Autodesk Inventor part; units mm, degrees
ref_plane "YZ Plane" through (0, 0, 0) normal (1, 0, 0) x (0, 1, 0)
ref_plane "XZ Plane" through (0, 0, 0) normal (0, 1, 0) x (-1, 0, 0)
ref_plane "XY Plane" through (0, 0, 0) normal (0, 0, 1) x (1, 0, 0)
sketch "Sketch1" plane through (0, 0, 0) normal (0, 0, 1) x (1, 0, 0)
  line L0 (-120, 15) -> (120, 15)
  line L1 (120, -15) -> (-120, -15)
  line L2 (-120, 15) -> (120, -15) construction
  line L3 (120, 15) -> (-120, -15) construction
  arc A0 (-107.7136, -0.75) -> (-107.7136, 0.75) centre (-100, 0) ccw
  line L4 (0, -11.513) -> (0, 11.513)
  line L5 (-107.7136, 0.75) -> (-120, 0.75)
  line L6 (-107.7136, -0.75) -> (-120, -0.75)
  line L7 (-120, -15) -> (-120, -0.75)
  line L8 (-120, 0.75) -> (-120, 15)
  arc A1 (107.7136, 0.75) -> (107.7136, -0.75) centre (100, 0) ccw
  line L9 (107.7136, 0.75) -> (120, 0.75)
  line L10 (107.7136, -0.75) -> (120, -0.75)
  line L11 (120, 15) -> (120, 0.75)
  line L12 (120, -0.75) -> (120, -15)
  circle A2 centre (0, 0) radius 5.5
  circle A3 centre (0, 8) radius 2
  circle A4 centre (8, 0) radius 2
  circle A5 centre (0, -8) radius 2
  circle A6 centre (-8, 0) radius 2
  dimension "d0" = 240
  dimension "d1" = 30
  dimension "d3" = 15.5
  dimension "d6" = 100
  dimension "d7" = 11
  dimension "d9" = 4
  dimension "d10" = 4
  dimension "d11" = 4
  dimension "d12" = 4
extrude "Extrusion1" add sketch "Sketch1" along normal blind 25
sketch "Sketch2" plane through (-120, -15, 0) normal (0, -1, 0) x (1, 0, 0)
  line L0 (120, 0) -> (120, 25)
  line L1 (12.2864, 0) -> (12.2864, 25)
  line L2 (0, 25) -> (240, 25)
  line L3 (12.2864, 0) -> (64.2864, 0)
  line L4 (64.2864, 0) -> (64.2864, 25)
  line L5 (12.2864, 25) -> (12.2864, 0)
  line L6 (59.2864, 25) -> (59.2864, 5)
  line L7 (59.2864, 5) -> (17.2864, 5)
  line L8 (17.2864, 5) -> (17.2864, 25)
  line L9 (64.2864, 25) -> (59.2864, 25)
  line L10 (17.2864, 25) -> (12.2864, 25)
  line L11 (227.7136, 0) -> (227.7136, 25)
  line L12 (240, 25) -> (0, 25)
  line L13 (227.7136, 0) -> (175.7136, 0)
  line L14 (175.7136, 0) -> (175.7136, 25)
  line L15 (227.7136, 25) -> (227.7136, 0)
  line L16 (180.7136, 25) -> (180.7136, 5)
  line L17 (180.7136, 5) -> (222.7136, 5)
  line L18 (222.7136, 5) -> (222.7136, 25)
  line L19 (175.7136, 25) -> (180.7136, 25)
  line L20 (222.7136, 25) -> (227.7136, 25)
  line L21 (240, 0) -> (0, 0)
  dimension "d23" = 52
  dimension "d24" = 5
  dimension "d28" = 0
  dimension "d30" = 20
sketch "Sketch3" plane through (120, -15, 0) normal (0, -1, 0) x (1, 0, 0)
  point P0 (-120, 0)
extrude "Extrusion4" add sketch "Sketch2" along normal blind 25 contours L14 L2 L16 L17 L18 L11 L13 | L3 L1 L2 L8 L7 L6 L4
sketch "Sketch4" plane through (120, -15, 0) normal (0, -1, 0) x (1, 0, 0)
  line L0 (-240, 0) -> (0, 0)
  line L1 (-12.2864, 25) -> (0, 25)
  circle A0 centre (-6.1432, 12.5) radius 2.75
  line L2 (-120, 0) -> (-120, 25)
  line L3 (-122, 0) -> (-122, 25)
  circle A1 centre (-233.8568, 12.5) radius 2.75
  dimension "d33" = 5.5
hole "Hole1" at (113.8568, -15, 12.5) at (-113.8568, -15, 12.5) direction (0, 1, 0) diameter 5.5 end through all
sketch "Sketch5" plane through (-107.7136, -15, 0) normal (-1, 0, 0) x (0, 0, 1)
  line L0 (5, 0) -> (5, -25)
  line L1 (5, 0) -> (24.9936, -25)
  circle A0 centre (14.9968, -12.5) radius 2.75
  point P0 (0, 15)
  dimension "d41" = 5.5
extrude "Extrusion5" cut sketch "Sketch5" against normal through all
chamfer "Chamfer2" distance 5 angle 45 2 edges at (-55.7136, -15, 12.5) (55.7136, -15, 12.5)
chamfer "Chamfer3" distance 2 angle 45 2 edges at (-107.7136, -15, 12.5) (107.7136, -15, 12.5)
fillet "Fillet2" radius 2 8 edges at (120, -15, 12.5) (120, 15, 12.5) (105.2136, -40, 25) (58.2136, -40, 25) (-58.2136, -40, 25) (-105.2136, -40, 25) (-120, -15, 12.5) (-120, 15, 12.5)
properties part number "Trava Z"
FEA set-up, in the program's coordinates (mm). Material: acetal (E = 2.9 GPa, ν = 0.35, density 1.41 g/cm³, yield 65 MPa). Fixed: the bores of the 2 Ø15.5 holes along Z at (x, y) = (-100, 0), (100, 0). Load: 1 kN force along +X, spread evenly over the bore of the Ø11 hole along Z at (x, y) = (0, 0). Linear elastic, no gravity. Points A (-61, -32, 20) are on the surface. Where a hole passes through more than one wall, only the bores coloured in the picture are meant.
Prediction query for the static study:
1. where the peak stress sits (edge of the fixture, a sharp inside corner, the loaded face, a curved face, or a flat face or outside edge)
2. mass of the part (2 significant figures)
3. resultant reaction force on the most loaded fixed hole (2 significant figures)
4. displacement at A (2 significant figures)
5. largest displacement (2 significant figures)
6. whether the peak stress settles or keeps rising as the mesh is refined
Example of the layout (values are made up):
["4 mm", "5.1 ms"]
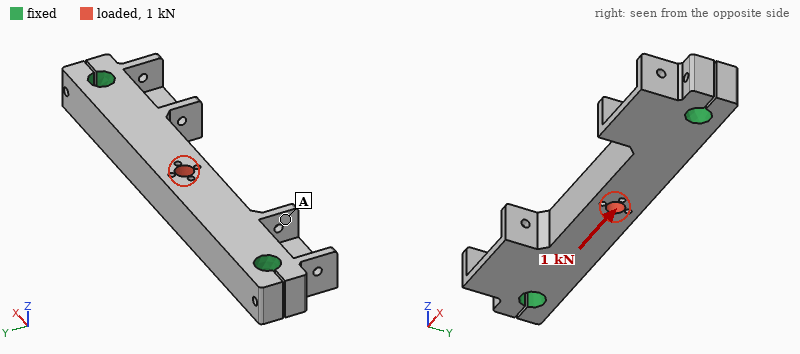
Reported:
["a sharp inside corner", "260 g", "500 N", "8.2 µm", "29 µm", "keeps rising"]
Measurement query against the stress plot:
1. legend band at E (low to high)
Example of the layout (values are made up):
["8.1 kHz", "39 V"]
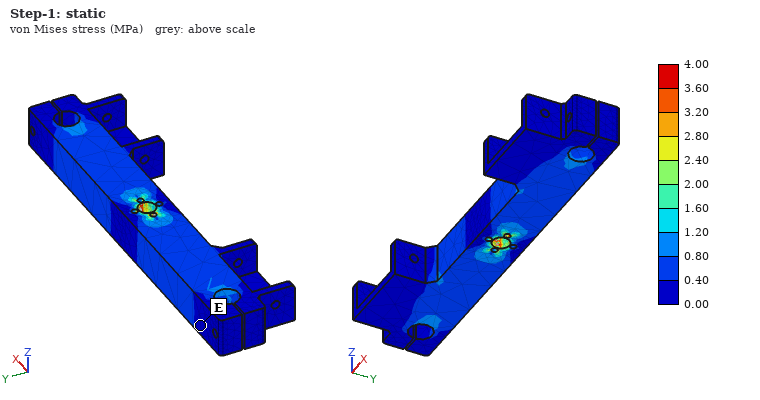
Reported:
["0.00 to 0.40 MPa"]
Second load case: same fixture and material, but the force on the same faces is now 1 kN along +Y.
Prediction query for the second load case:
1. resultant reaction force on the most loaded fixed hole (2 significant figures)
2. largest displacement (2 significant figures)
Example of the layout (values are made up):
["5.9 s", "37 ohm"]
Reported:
["500 N", "0.33 mm"]
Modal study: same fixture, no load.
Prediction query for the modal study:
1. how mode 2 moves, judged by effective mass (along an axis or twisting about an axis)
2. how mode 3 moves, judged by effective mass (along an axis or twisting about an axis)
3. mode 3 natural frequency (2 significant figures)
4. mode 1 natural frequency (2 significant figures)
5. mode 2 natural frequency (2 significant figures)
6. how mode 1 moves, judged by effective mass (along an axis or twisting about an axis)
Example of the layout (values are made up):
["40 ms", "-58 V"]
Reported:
["along Y", "twisting about X", "1800 Hz", "900 Hz", "1000 Hz", "along Z"]
